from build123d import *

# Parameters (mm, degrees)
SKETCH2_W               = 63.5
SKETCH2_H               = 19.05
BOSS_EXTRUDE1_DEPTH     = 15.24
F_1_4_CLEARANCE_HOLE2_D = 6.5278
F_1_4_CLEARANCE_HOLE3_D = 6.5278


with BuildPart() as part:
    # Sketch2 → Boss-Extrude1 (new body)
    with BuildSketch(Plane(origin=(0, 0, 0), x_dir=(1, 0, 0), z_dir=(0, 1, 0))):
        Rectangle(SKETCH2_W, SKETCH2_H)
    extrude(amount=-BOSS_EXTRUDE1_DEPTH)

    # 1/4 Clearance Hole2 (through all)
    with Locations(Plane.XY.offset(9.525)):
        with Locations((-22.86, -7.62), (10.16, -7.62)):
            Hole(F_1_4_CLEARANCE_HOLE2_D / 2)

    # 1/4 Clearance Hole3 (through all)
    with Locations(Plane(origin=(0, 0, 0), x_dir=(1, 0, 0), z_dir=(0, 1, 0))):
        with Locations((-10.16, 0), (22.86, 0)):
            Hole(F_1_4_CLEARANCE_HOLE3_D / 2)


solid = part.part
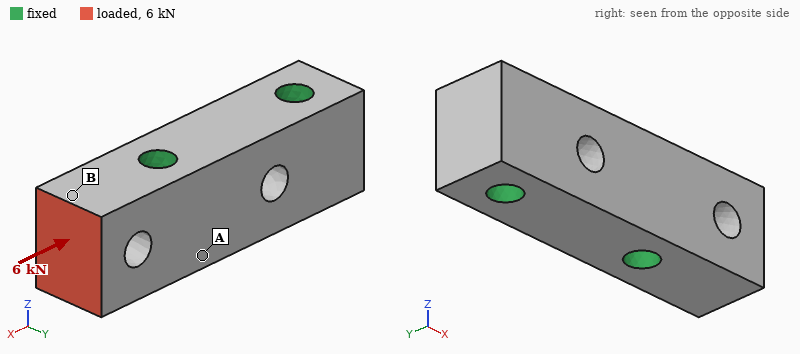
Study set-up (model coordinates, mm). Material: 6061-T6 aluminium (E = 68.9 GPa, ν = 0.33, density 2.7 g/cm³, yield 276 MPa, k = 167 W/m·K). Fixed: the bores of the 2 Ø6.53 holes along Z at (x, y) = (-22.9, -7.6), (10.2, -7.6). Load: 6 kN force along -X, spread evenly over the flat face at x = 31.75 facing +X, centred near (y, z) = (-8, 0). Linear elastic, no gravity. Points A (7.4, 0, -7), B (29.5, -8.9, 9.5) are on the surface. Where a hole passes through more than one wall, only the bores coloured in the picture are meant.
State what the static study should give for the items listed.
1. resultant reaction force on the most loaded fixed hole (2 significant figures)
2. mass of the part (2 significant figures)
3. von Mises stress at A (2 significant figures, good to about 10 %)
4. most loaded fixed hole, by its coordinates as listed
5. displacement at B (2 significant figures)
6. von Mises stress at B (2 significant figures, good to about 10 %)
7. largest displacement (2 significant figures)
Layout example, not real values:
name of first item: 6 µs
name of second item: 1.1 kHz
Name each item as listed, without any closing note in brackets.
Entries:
resultant reaction force on the most loaded fixed hole: 5.8 kN
mass of the part: 44 g
von Mises stress at A: 8.3 MPa
most loaded fixed hole, by its coordinates as listed: (10.2, -7.6)
displacement at B: 6.1 µm
von Mises stress at B: 20 MPa
largest displacement: 9.6 µm
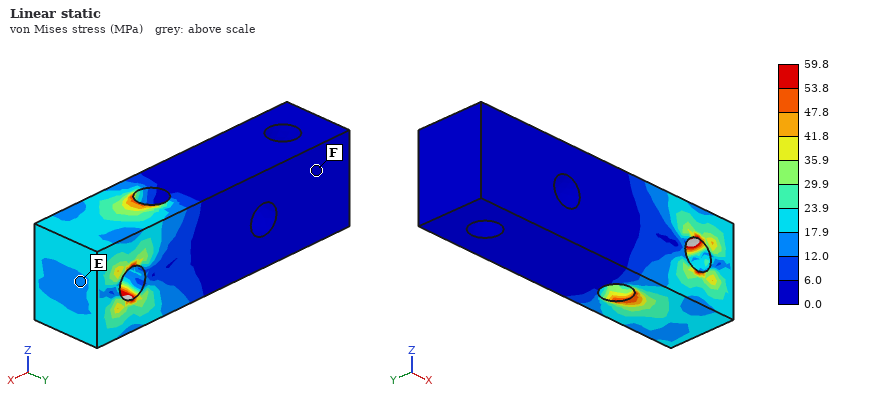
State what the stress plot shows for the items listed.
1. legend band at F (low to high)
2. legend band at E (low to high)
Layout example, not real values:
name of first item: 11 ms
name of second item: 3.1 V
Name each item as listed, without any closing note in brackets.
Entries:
legend band at F: 0.0 to 6.0 MPa
legend band at E: 12.0 to 17.9 MPa
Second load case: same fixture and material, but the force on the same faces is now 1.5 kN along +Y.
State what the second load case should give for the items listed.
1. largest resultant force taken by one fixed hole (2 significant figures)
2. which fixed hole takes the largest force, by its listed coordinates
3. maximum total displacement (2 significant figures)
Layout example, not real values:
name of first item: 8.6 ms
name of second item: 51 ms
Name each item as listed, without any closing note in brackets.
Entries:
largest resultant force taken by one fixed hole: 1.8 kN
which fixed hole takes the largest force, by its listed coordinates: (10.2, -7.6)
maximum total displacement: 26 µm
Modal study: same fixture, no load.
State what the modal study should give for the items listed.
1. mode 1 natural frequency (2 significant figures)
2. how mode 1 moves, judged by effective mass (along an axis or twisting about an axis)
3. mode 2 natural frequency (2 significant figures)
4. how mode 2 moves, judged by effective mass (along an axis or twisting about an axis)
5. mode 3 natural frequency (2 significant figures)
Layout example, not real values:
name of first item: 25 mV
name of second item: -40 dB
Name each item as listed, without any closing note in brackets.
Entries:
mode 1 natural frequency: 19 kHz
how mode 1 moves, judged by effective mass: along Y
mode 2 natural frequency: 23 kHz
how mode 2 moves, judged by effective mass: along Z
mode 3 natural frequency: 32 kHz
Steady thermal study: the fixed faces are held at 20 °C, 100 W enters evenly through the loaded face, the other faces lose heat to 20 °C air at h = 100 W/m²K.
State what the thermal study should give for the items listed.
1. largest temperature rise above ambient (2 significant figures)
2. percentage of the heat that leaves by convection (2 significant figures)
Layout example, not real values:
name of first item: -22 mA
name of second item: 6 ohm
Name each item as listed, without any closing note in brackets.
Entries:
largest temperature rise above ambient: 49 K
percentage of the heat that leaves by convection: 3.9 %
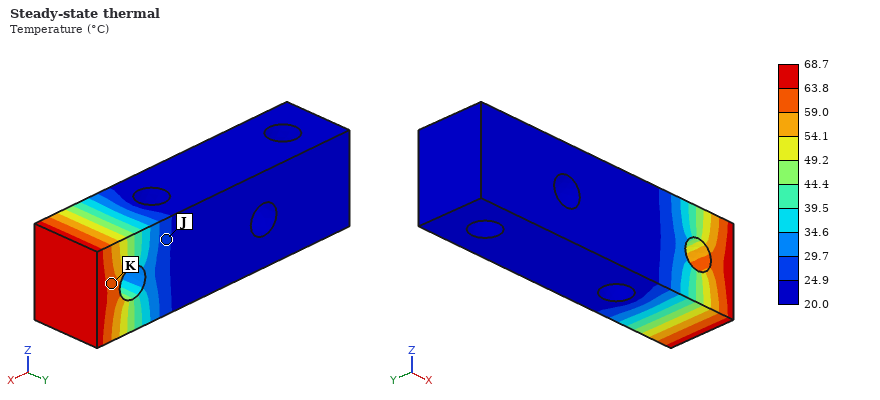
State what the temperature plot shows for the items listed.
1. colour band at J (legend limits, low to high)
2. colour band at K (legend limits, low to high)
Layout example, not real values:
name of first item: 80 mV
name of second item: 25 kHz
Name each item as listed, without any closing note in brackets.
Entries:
colour band at J: 24.9 to 29.7 °C
colour band at K: 59.0 to 63.8 °C
